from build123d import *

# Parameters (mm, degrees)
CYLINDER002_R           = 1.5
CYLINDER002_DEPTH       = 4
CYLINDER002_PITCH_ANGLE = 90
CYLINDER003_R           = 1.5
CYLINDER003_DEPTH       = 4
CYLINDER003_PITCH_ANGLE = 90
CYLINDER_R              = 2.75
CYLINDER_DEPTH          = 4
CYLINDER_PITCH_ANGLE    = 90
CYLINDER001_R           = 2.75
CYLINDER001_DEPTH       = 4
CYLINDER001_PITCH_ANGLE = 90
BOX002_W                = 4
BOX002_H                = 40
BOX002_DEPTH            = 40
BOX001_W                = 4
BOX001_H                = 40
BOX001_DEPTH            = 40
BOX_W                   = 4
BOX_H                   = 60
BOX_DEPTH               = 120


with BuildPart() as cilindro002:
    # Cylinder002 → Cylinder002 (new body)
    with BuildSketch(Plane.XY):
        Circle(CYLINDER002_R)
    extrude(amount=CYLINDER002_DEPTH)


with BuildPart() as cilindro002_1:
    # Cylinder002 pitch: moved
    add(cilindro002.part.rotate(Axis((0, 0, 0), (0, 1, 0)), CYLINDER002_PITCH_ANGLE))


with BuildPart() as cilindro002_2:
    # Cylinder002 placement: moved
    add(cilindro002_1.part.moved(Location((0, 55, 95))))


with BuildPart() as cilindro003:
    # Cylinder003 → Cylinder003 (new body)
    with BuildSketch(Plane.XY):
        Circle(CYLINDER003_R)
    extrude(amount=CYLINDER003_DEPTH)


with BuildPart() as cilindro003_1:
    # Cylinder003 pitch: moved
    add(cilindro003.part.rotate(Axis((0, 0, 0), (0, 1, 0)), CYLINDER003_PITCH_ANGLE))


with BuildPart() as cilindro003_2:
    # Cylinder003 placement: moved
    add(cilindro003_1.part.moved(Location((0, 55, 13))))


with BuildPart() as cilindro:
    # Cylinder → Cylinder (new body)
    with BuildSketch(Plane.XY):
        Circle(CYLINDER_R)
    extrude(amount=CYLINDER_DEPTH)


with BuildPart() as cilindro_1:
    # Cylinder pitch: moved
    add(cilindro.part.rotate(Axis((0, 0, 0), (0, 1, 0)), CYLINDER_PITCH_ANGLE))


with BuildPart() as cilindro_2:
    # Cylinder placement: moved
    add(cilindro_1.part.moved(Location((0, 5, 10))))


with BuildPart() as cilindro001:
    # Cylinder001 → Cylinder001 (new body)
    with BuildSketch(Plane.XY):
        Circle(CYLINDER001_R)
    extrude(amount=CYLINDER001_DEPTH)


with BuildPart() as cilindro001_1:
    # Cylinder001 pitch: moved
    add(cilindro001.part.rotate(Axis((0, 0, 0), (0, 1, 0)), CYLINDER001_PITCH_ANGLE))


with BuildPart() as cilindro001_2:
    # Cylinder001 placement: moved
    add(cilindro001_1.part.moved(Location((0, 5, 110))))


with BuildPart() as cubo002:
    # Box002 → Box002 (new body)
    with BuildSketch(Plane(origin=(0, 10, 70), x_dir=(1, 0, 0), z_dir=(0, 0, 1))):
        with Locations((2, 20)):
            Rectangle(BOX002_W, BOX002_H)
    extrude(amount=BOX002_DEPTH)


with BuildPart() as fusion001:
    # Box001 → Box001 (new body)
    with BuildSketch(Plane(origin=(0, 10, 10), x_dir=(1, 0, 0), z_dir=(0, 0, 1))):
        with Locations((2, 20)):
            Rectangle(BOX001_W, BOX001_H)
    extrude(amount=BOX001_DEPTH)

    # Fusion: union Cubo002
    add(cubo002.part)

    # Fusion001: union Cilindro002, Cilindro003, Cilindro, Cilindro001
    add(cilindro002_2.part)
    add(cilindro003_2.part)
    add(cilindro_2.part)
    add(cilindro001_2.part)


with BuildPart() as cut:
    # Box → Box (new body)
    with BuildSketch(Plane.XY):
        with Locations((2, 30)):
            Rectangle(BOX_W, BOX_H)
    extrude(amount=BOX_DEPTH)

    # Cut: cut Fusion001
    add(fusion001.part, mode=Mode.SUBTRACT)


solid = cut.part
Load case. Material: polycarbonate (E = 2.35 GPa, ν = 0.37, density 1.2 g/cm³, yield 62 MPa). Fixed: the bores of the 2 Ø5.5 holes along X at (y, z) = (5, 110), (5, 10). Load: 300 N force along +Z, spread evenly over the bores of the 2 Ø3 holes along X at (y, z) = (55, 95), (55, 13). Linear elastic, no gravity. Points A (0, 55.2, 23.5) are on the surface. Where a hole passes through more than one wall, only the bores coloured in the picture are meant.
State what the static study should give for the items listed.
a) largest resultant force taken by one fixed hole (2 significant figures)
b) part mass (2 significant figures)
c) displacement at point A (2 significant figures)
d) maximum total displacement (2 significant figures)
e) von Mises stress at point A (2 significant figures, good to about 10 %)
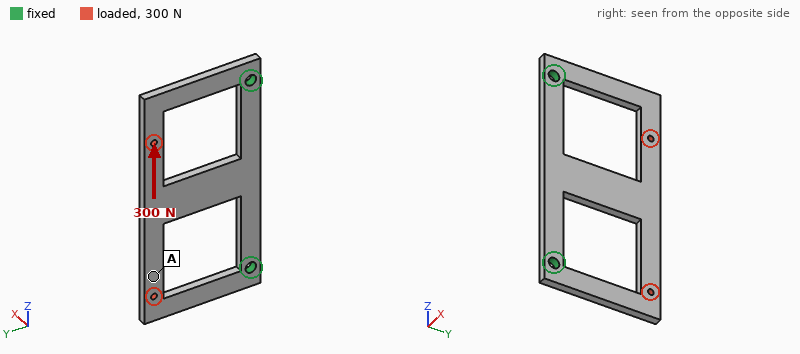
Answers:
200 N
19 g
1.3 mm
1.4 mm
5.1 MPa
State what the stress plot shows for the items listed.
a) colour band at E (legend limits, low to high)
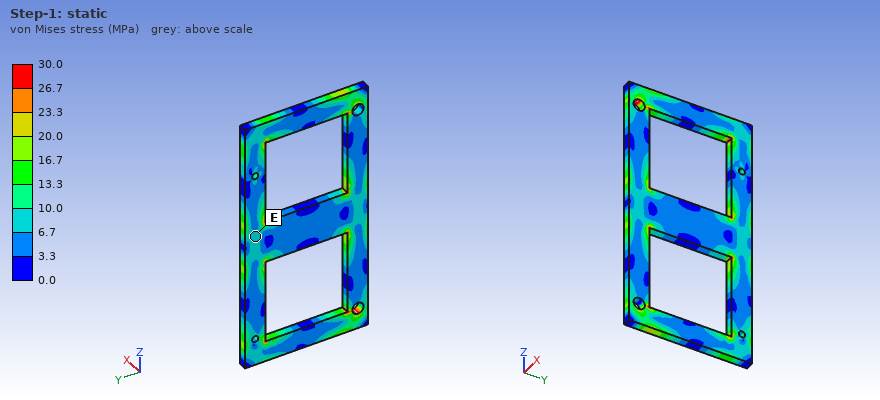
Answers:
6.7 to 10.0 MPa
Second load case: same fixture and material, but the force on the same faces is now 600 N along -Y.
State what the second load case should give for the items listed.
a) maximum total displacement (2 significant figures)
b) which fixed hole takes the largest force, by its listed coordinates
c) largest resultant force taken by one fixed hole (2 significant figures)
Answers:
0.90 mm
(5, 10)
340 N
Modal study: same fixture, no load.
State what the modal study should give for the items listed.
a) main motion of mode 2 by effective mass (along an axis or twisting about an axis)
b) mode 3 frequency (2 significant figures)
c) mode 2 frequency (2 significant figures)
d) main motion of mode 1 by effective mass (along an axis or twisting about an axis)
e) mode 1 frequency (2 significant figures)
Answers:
twisting about Y
460 Hz
320 Hz
along X
160 Hz
